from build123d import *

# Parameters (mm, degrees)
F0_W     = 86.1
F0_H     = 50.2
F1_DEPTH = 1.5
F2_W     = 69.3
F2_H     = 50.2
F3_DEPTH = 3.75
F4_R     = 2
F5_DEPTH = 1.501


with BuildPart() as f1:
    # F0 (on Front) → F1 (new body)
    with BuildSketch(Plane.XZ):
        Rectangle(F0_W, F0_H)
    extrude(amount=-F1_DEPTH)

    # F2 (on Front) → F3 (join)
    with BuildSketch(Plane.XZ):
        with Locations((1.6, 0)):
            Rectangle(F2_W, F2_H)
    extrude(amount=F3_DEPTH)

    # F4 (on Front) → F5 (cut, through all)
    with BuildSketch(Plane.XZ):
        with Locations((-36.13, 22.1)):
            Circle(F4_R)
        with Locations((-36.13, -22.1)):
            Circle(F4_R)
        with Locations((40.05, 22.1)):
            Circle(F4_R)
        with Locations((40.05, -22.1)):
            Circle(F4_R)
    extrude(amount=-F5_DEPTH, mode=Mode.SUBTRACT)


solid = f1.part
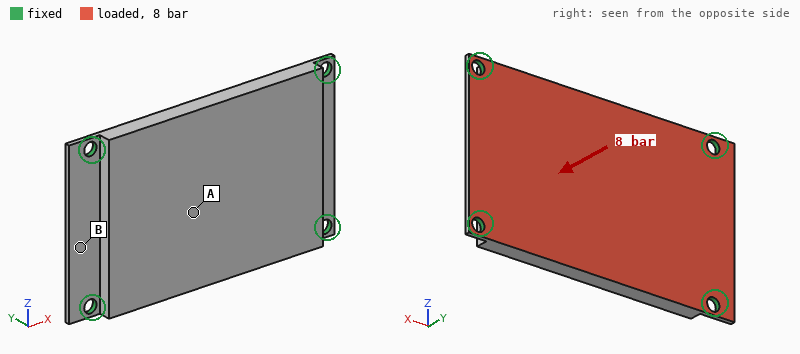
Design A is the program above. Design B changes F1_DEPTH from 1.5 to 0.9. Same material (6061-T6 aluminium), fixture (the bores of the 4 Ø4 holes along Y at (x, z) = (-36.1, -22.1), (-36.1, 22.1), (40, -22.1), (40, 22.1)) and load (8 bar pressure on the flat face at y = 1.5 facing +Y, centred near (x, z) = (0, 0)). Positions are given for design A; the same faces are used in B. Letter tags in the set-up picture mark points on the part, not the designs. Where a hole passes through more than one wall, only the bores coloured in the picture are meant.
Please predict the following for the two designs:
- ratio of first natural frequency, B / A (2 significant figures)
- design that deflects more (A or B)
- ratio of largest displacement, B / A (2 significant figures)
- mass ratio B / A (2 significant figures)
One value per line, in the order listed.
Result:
0.86
B
1.5
0.87
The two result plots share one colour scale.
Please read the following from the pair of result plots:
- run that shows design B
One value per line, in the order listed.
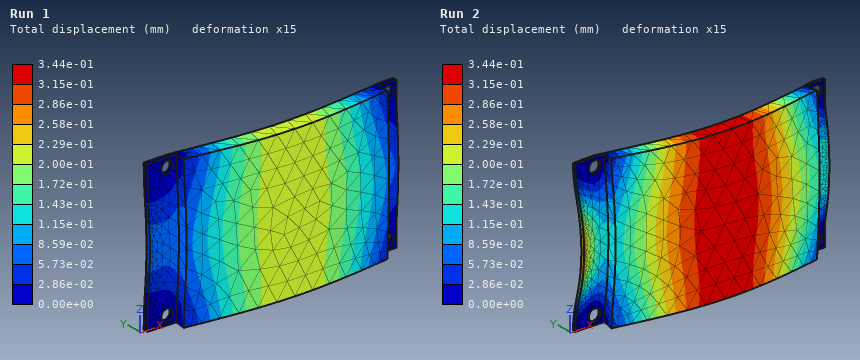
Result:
Run 2
